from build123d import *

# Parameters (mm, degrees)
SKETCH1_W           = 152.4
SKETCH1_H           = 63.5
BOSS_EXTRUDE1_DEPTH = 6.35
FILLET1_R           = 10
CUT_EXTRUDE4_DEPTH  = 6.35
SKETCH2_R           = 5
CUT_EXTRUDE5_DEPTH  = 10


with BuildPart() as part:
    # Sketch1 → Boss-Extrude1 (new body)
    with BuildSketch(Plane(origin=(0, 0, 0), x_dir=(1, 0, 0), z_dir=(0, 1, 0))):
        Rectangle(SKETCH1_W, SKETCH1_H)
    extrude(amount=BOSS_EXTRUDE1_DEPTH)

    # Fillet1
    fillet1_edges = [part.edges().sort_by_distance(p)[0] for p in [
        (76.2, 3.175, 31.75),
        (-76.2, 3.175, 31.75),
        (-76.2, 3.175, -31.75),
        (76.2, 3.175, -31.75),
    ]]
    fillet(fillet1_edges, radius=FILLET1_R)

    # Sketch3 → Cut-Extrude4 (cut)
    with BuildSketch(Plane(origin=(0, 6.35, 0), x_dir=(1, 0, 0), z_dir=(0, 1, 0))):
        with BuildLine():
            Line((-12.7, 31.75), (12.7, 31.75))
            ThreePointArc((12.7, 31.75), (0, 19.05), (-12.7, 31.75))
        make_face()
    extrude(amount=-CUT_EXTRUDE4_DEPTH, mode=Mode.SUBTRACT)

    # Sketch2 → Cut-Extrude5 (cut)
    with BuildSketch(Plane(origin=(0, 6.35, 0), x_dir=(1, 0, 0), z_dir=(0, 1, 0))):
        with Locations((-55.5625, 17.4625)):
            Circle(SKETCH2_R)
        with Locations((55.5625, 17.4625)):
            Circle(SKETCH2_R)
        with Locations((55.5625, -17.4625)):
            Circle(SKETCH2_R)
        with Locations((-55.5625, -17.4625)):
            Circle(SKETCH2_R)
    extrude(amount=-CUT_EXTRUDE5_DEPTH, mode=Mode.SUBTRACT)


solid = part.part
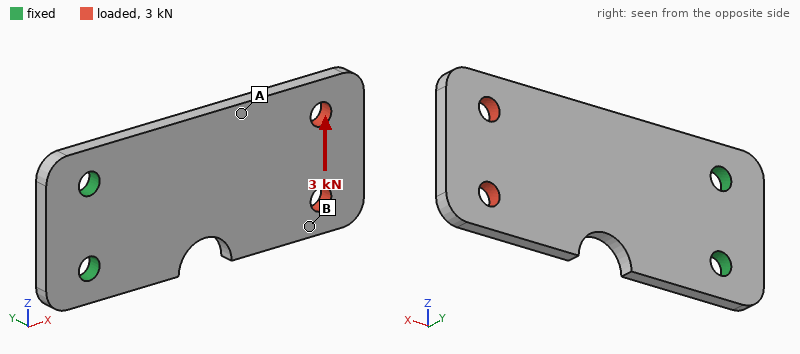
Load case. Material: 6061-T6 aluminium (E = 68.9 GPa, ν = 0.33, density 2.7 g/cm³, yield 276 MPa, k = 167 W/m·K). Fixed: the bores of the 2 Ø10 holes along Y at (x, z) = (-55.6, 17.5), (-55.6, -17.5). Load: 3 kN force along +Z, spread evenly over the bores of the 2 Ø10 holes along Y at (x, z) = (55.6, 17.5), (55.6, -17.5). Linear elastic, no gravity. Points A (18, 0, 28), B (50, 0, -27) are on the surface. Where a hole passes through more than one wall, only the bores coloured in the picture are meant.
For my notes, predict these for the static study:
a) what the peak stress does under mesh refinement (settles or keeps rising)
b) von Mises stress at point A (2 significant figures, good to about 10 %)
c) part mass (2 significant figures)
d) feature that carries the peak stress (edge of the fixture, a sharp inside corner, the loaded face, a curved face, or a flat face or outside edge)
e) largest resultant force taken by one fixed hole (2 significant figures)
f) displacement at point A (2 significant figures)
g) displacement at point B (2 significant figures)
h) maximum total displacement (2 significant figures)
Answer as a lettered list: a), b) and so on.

a) keeps rising
b) 32 MPa
c) 150 g
d) edge of the fixture
e) 8.3 kN
f) 0.13 mm
g) 0.23 mm
h) 0.30 mm
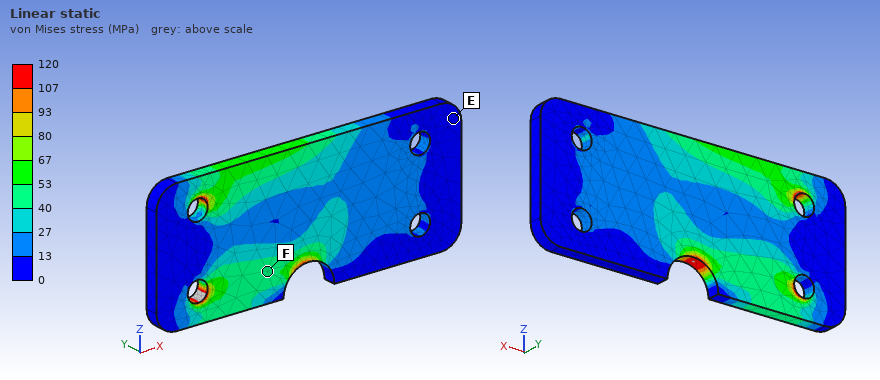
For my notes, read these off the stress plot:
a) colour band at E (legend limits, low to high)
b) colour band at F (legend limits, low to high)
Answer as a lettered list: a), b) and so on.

a) 0 to 13 MPa
b) 40 to 53 MPa
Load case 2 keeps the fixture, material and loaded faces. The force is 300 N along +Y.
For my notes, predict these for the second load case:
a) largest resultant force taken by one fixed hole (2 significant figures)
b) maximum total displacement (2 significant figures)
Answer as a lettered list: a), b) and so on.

a) 150 N
b) 1.8 mm
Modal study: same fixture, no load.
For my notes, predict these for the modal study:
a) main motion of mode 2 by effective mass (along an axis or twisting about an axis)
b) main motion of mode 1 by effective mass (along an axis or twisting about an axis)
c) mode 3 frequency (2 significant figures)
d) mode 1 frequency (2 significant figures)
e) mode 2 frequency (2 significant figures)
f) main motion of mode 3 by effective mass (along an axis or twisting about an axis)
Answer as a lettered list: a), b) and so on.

a) twisting about X
b) along Y
c) 1900 Hz
d) 320 Hz
e) 1300 Hz
f) along Y
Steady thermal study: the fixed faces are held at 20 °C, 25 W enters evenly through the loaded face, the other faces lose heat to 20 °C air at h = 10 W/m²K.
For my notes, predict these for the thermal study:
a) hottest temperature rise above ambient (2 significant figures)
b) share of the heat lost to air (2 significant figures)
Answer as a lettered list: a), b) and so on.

a) 41 K
b) 16 %
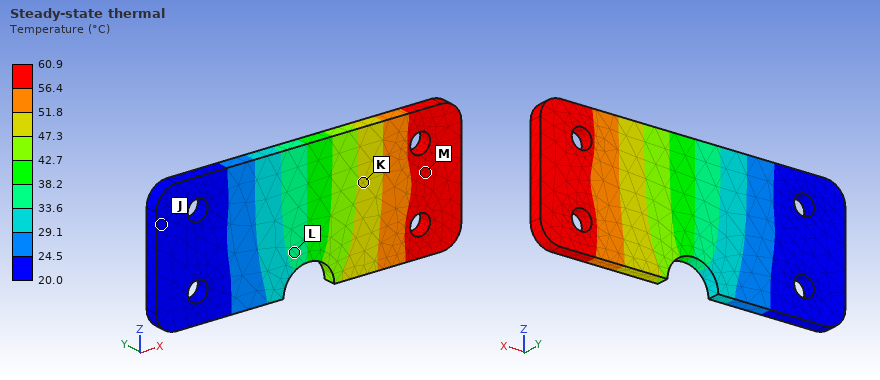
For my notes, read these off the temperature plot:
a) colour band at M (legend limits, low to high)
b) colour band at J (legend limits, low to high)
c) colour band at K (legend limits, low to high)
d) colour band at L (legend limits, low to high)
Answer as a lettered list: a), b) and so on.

a) 56.4 to 60.9 °C
b) 20.0 to 24.5 °C
c) 47.3 to 51.8 °C
d) 33.6 to 38.2 °C
